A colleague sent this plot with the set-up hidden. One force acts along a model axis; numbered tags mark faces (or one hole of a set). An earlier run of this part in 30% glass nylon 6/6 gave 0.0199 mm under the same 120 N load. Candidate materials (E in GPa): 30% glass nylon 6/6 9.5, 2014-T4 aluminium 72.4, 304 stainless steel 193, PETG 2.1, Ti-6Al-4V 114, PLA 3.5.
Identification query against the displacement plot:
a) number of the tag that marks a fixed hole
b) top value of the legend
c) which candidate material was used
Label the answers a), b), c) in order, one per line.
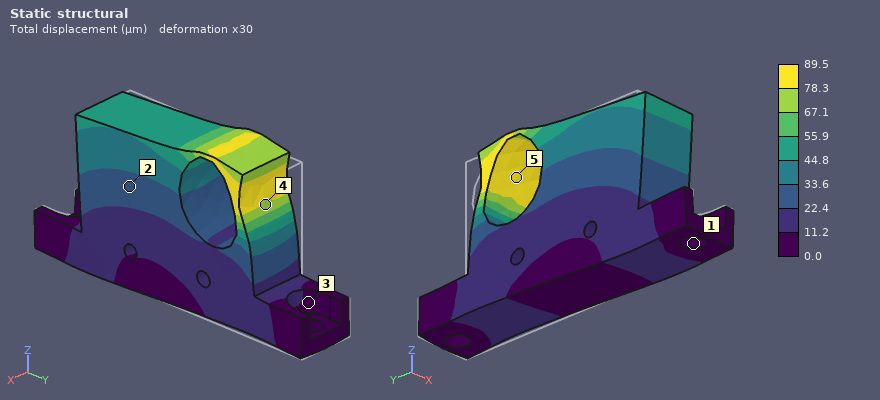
a) 1
b) 89.5 µm
c) PETG
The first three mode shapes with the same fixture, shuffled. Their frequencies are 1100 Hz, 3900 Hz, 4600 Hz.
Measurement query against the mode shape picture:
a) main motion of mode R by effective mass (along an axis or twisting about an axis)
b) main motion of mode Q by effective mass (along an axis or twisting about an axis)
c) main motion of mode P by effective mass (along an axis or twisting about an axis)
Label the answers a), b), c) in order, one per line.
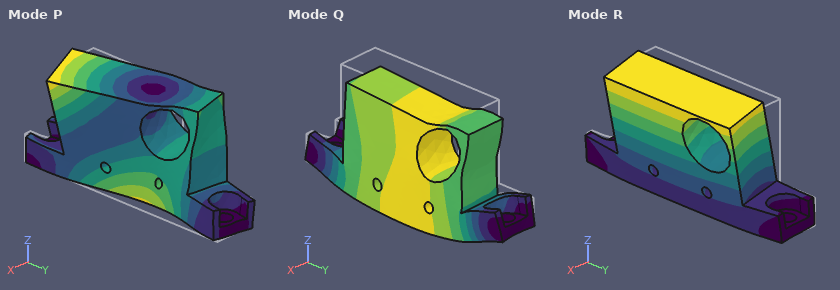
a) along X
b) along Z
c) along X
